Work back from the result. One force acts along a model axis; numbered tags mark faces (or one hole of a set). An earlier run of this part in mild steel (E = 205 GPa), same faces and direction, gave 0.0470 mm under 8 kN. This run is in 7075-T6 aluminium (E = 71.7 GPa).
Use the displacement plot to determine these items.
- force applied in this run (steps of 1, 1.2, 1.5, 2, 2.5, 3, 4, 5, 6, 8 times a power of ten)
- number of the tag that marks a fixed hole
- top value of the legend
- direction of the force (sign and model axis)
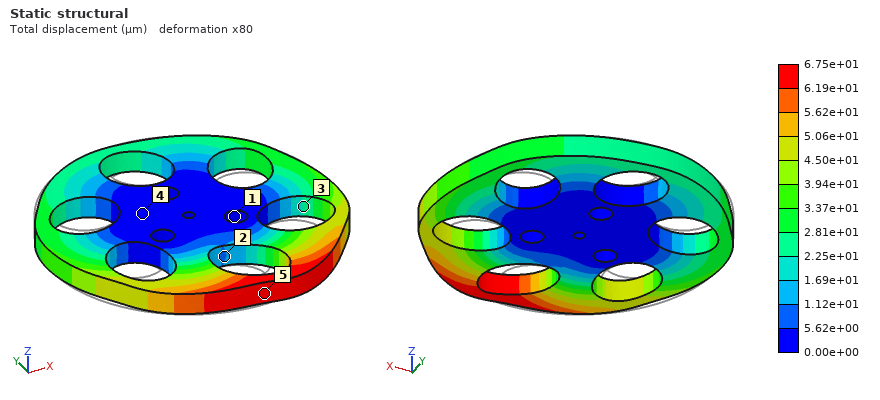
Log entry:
4 kN
1
6.75e+01 µm
+X
